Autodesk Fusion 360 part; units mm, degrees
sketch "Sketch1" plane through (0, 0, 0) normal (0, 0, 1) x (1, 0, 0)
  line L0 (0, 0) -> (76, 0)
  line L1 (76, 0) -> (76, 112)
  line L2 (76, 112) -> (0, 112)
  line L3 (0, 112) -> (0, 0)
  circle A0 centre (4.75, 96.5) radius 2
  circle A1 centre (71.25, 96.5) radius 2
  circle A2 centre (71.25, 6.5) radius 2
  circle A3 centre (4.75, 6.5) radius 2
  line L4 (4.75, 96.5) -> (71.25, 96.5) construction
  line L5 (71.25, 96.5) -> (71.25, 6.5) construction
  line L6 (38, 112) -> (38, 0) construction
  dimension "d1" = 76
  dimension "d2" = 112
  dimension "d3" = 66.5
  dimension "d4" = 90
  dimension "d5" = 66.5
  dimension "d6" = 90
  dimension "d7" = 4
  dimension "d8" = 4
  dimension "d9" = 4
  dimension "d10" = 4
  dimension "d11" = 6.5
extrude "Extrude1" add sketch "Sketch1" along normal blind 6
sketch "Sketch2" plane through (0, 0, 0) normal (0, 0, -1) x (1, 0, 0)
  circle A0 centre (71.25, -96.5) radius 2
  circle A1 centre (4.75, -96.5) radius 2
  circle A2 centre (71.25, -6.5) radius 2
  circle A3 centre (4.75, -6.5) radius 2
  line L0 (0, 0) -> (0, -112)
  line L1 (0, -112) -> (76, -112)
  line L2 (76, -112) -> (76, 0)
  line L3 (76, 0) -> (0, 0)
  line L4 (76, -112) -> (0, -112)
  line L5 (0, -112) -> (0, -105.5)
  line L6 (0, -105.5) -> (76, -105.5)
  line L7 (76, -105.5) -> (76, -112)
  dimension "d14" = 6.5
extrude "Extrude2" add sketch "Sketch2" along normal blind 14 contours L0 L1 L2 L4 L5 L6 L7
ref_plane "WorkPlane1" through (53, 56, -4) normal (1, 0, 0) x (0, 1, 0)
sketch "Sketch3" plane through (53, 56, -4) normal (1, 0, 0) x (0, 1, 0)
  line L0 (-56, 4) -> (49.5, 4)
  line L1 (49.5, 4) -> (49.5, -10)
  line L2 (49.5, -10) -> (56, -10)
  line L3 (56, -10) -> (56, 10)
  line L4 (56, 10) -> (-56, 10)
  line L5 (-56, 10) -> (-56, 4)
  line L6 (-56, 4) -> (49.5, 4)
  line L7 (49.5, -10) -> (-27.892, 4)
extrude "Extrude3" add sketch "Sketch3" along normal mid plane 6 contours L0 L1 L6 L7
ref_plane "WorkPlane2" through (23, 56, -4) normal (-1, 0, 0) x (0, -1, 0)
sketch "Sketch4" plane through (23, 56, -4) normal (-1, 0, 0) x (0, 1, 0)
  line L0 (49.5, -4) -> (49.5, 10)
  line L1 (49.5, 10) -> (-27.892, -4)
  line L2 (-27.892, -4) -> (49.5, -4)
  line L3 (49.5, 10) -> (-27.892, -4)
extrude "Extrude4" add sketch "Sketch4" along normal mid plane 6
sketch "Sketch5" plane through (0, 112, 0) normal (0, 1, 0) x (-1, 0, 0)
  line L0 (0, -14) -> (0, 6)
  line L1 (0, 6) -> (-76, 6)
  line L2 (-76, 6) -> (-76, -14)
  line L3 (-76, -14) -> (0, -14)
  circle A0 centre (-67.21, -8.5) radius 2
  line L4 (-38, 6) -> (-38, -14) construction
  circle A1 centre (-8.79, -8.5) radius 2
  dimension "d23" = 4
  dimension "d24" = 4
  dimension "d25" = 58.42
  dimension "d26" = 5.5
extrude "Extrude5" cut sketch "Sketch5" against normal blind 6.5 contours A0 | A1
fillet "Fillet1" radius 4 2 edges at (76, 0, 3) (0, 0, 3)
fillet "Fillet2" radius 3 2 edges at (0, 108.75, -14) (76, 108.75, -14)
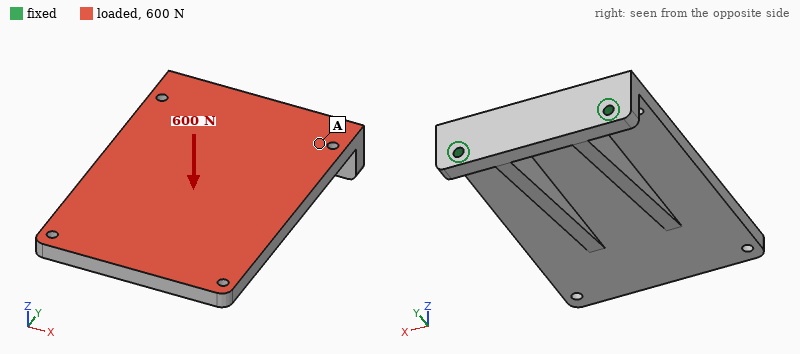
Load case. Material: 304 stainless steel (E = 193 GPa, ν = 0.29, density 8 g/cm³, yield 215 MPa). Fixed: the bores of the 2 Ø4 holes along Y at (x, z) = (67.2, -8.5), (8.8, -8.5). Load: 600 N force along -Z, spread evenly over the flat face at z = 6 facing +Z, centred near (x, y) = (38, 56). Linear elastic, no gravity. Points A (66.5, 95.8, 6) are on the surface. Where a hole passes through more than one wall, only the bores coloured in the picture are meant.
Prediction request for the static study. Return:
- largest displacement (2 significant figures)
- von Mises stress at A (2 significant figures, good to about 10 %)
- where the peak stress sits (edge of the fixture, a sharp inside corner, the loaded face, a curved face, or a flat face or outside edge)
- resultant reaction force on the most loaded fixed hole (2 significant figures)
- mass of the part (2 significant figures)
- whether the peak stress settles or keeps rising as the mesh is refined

0.22 mm
14 MPa
edge of the fixture
370 N
510 g
keeps rising
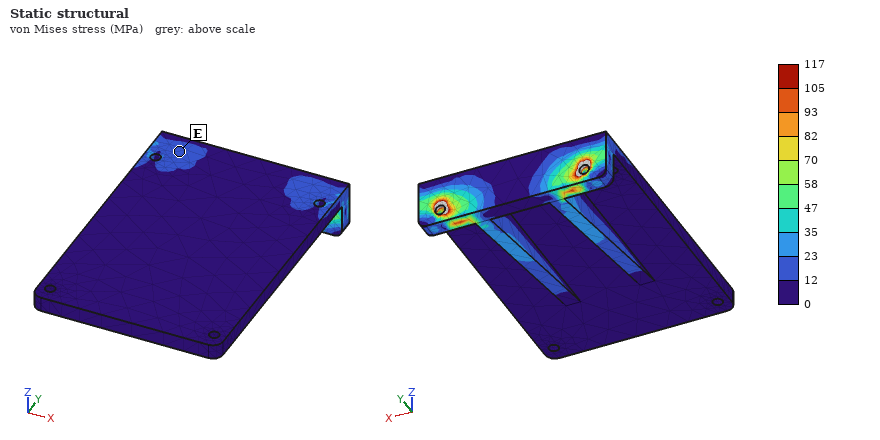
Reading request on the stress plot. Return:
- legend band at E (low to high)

12 to 23 MPa
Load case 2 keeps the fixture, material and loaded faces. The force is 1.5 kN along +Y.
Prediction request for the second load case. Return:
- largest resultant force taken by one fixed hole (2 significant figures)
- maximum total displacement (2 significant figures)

750 N
98 µm
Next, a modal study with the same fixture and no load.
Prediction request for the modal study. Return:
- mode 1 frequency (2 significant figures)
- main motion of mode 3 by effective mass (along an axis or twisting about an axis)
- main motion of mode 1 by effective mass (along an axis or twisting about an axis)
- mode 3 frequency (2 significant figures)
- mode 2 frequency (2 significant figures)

510 Hz
along X
along Z
2200 Hz
1400 Hz
